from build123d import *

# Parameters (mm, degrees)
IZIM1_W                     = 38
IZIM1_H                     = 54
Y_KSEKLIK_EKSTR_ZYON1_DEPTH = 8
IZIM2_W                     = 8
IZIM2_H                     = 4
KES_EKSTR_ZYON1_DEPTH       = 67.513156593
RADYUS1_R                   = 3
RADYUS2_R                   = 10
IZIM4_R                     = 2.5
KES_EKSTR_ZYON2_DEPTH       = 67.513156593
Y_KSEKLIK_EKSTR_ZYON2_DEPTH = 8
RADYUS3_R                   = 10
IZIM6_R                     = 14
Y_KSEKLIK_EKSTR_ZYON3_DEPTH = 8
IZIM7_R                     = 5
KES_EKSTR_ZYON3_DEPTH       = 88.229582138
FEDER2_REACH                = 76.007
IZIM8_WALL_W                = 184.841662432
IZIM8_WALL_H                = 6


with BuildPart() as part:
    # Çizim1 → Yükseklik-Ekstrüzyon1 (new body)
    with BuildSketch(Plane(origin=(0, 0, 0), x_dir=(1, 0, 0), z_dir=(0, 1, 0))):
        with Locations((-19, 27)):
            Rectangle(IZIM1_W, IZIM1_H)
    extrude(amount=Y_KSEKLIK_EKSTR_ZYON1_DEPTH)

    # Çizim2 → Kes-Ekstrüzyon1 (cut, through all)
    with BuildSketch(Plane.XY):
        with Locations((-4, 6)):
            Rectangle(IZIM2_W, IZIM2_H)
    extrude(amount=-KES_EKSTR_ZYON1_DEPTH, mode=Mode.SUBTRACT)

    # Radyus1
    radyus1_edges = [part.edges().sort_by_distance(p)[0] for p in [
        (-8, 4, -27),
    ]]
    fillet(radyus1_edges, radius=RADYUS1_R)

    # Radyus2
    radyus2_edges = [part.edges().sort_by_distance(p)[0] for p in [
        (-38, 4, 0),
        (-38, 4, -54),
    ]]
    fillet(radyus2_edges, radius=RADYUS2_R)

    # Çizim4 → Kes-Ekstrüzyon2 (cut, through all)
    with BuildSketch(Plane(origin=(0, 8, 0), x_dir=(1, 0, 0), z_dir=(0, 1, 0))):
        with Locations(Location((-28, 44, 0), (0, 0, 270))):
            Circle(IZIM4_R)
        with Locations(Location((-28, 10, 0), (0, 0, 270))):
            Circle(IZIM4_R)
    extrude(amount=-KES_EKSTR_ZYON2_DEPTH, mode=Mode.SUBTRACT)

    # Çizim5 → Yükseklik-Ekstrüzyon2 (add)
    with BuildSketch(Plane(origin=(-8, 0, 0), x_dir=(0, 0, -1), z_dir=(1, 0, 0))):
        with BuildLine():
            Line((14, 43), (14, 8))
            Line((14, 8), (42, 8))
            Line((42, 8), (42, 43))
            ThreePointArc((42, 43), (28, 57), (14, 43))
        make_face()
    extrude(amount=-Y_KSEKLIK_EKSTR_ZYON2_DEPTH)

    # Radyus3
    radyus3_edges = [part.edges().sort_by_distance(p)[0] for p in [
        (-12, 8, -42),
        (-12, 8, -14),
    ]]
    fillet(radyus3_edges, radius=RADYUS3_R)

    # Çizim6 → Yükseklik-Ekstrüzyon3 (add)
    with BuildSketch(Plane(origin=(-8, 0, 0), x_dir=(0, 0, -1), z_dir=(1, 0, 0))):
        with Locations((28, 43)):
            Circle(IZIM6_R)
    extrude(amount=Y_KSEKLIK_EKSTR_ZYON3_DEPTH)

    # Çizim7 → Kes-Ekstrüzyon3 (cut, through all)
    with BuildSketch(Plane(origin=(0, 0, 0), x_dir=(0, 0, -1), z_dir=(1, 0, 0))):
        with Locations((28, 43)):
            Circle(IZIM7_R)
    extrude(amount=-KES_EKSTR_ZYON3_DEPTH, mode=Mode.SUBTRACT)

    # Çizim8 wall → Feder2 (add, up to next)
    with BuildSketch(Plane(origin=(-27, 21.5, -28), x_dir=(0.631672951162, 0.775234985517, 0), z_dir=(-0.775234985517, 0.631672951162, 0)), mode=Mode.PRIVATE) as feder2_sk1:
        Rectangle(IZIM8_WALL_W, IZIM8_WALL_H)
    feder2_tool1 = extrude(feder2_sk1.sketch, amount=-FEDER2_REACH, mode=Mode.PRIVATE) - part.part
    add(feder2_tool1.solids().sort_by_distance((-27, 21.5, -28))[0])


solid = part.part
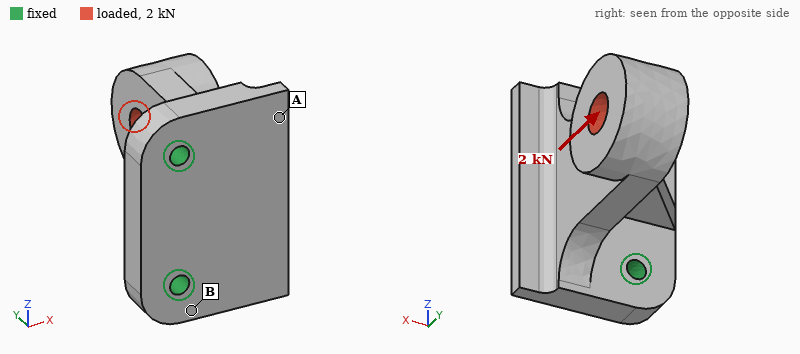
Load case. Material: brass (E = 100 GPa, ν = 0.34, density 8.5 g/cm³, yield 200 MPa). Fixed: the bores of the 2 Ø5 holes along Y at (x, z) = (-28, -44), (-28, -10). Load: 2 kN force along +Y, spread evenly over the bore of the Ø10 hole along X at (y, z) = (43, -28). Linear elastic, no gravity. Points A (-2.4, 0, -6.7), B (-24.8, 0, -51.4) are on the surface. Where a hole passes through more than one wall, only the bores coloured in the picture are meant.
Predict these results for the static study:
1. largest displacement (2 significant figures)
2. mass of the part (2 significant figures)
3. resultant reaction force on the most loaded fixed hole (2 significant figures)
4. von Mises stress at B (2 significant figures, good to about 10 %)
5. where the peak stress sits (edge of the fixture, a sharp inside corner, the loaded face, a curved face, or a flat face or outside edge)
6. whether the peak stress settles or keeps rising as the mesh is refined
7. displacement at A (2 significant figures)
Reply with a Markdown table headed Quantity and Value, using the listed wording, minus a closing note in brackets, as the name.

| Quantity | Value |
|---|---|
| largest displacement | 0.11 mm |
| mass of the part | 260 g |
| resultant reaction force on the most loaded fixed hole | 1.1 kN |
| von Mises stress at B | 33 MPa |
| where the peak stress sits | edge of the fixture |
| whether the peak stress settles or keeps rising as the mesh is refined | keeps rising |
| displacement at A | 0.033 mm |
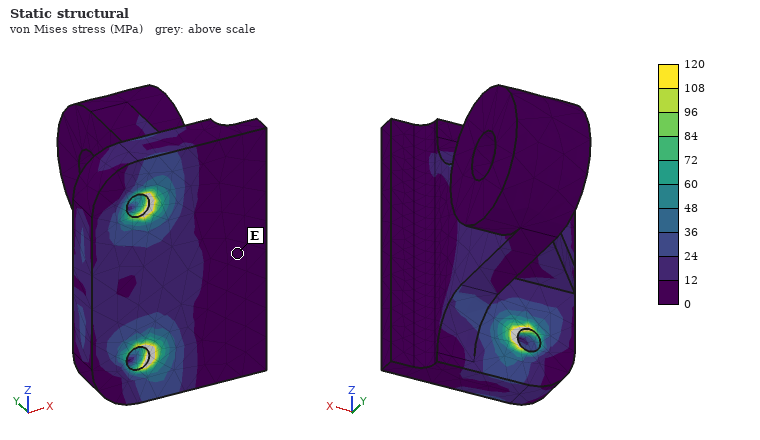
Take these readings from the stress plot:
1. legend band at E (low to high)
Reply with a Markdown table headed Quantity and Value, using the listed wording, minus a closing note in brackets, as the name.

| Quantity | Value |
|---|---|
| legend band at E | 0 to 12 MPa |
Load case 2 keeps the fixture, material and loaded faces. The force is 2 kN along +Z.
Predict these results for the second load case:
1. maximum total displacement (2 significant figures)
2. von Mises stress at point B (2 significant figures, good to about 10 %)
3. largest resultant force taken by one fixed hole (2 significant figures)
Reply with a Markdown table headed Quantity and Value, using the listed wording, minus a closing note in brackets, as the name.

| Quantity | Value |
|---|---|
| maximum total displacement | 100 µm |
| von Mises stress at point B | 38 MPa |
| largest resultant force taken by one fixed hole | 2.7 kN |
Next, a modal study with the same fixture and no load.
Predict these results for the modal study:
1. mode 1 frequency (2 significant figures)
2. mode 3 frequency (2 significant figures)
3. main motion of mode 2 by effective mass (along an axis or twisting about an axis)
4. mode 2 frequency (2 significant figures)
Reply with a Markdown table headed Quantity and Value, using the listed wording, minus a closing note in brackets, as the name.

| Quantity | Value |
|---|---|
| mode 1 frequency | 1600 Hz |
| mode 3 frequency | 5500 Hz |
| main motion of mode 2 by effective mass | along Z |
| mode 2 frequency | 2800 Hz |
